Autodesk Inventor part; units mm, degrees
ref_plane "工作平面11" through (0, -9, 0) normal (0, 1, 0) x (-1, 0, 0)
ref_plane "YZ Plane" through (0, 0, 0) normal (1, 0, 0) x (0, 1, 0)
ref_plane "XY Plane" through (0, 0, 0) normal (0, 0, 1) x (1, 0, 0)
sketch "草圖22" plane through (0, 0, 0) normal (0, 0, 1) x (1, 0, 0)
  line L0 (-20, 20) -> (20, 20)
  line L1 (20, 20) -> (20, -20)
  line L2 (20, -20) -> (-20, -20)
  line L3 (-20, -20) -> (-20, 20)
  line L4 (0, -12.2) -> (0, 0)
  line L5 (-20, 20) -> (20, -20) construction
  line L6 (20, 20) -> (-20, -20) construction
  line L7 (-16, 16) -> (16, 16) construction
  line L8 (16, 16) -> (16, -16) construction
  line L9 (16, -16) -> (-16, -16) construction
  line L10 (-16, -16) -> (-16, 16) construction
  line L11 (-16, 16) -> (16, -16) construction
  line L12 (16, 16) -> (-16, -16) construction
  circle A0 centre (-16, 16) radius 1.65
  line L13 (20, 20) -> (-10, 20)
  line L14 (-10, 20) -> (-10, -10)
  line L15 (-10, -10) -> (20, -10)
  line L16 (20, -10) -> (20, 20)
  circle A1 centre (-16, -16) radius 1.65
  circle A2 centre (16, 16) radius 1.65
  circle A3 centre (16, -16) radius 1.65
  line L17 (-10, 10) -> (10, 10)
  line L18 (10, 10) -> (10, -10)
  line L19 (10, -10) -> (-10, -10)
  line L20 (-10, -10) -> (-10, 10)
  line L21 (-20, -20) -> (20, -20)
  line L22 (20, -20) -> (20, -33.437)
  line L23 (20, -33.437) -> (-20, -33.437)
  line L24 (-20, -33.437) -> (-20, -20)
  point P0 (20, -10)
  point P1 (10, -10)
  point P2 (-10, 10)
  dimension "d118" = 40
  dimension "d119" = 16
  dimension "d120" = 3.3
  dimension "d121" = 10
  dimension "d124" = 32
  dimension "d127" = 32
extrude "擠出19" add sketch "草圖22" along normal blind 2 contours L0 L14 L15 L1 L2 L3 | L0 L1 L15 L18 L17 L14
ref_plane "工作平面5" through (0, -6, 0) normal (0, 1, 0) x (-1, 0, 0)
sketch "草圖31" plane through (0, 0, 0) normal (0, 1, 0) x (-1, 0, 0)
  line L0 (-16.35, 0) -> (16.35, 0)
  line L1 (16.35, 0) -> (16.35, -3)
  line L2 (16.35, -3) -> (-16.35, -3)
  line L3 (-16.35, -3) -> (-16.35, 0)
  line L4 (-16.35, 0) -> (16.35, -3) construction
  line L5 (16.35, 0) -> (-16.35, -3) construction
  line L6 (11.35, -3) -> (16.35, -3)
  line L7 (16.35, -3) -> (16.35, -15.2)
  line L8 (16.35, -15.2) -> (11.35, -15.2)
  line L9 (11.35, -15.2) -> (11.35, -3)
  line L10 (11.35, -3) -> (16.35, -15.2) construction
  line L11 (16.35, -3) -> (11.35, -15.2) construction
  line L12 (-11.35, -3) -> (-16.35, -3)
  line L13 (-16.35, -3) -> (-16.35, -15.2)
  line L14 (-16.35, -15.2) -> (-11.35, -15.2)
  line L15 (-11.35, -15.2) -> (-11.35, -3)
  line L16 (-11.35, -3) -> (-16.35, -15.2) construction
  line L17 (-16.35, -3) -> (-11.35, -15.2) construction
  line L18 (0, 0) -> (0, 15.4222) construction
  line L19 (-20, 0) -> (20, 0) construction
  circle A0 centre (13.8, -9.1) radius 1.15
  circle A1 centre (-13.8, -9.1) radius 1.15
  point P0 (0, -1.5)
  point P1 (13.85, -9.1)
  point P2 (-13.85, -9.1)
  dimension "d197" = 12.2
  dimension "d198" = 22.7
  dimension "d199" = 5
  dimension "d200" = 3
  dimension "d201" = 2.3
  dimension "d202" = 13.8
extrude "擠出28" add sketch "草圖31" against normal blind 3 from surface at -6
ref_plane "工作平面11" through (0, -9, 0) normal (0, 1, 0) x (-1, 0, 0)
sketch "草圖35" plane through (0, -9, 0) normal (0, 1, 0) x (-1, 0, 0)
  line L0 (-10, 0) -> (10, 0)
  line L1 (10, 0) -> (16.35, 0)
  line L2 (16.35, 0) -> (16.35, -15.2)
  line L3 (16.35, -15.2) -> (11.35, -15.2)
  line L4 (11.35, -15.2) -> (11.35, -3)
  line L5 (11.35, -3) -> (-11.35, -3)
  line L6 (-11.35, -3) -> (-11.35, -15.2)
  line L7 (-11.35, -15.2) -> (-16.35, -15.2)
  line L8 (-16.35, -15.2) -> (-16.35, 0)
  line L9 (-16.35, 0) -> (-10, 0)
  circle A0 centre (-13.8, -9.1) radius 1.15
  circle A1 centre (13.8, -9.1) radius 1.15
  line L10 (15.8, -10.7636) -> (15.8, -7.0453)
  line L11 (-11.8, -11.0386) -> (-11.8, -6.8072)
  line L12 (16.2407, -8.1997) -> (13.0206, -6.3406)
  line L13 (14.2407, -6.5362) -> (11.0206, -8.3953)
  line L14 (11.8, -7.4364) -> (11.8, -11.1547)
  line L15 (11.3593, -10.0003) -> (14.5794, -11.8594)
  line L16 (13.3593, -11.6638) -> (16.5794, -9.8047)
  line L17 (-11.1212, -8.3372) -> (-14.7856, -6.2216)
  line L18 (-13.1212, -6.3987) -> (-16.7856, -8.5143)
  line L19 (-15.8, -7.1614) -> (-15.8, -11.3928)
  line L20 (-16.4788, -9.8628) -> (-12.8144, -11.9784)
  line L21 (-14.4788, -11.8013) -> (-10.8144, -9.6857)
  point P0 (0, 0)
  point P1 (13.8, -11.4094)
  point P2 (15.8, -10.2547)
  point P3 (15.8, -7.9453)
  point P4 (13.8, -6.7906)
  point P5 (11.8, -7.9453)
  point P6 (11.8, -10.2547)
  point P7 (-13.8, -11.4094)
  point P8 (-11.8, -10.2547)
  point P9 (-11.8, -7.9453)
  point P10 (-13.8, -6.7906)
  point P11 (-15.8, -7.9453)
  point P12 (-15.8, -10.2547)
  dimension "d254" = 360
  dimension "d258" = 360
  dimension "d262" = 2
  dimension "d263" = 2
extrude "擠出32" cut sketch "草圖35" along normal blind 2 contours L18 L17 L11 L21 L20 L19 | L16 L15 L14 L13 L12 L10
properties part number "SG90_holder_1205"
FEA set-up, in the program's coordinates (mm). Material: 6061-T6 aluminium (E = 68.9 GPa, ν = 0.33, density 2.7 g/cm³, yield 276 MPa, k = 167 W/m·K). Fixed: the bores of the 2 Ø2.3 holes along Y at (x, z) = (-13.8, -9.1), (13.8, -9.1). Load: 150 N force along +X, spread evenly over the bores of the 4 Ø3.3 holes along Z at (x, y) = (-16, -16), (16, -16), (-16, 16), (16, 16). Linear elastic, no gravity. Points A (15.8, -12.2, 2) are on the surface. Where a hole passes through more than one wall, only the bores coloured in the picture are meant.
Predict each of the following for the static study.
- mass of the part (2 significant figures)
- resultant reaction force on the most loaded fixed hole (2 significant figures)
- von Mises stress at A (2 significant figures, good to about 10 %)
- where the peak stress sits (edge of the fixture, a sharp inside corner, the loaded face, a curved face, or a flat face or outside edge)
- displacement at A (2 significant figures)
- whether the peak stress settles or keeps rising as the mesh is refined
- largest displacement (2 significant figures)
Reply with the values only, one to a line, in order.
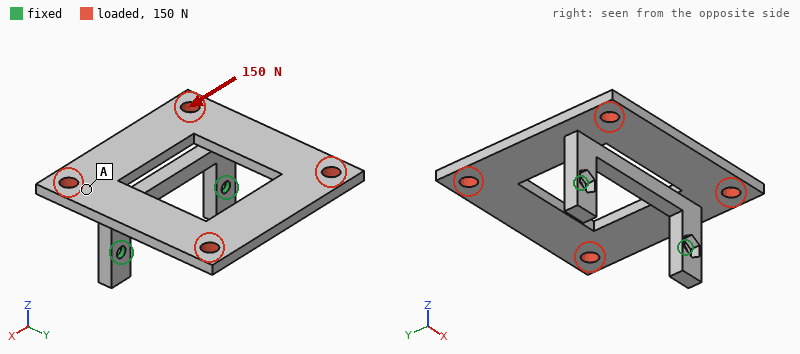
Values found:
7.9 g
86 N
8.6 MPa
edge of the fixture
27 µm
keeps rising
67 µm
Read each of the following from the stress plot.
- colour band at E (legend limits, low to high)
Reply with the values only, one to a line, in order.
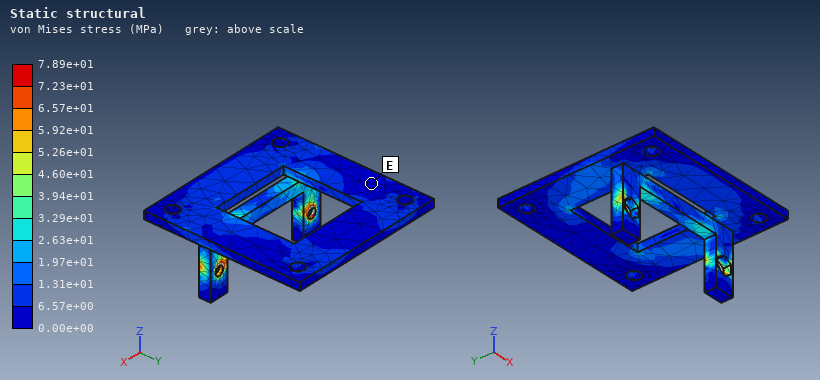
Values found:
0.00e+00 to 6.57e+00 MPa
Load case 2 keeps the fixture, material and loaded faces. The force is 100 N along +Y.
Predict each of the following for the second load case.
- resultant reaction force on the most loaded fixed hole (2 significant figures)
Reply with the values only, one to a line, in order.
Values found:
50 N
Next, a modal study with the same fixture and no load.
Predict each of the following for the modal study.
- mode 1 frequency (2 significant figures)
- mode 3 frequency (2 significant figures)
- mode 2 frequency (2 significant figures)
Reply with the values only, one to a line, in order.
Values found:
1000 Hz
3200 Hz
2500 Hz
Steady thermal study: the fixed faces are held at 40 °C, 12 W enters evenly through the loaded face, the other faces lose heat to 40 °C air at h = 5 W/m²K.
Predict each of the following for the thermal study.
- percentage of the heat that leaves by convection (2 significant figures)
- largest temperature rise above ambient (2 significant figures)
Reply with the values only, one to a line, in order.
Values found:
4.4 %
46 K
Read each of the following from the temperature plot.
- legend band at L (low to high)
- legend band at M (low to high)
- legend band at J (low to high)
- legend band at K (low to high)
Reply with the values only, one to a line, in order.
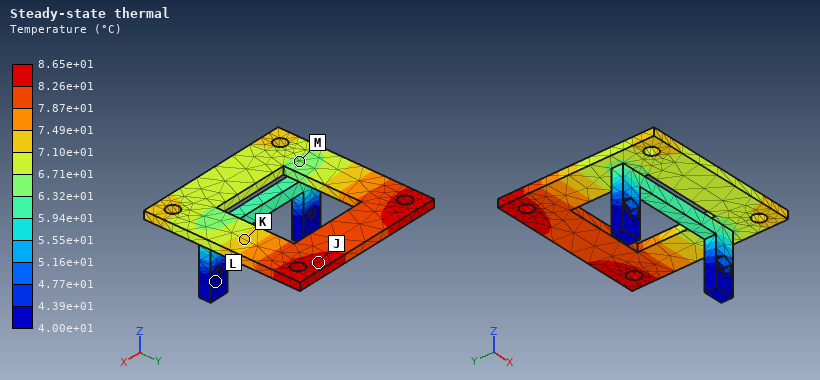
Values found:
4.00e+01 to 4.39e+01 °C
6.32e+01 to 6.71e+01 °C
8.26e+01 to 8.65e+01 °C
7.10e+01 to 7.49e+01 °C
